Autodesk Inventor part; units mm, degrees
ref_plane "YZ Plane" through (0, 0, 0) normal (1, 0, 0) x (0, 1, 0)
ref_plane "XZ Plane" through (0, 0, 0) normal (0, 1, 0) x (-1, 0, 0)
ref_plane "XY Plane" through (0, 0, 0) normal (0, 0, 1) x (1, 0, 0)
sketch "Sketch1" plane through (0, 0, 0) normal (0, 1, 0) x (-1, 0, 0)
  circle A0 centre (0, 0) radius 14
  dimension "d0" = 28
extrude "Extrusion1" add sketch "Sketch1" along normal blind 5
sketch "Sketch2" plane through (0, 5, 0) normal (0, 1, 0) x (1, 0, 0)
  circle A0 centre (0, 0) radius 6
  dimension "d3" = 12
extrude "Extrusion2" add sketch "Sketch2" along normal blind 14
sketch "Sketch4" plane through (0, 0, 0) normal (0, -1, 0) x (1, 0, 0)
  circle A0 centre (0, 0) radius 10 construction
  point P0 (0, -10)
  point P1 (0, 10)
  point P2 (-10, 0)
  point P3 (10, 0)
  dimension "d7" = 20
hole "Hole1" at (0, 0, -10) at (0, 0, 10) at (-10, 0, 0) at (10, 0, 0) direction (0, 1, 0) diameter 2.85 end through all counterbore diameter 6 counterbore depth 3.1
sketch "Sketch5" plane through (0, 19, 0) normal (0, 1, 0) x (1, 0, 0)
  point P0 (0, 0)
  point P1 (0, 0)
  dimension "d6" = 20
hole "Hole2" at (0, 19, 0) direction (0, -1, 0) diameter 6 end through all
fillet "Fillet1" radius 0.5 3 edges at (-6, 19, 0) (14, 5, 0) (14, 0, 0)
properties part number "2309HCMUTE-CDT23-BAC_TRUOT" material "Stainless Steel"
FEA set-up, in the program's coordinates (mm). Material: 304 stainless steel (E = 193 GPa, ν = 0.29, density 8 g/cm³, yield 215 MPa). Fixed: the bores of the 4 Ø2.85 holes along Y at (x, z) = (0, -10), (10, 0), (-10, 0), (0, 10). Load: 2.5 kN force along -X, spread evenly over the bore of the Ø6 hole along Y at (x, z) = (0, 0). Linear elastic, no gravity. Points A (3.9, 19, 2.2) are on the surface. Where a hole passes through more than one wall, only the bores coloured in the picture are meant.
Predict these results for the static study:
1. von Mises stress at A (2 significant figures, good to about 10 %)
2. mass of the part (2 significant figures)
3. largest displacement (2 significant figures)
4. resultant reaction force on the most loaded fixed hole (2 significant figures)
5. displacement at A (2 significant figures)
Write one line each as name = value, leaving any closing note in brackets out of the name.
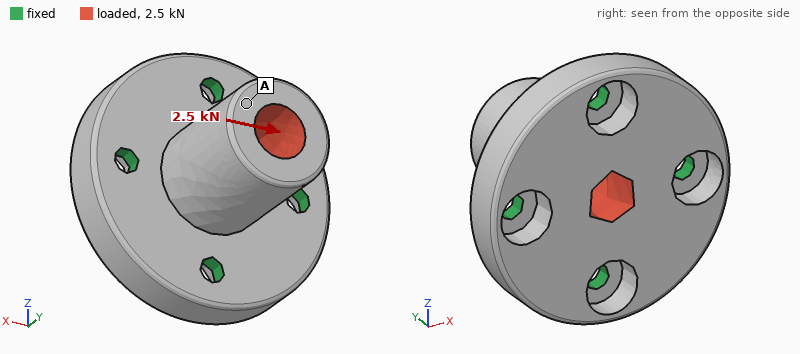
von Mises stress at A = 12 MPa
mass of the part = 30 g
largest displacement = 15 µm
resultant reaction force on the most loaded fixed hole = 960 N
displacement at A = 15 µm
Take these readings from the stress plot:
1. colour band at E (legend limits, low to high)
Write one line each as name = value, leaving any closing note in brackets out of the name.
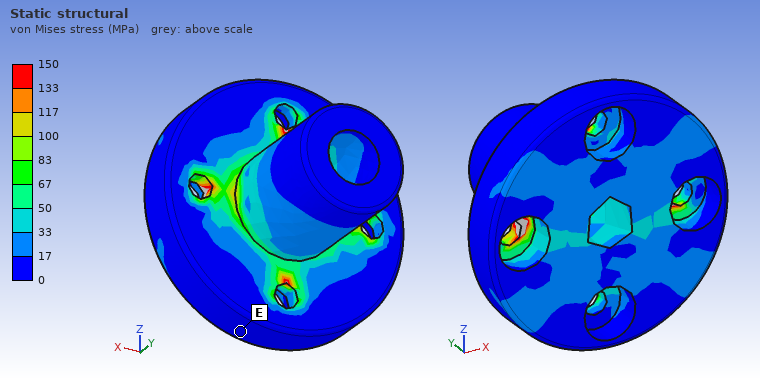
colour band at E = 0 to 17 MPa
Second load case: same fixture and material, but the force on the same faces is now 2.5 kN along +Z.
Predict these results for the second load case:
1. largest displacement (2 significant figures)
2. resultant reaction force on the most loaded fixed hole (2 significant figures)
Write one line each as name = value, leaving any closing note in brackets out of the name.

largest displacement = 15 µm
resultant reaction force on the most loaded fixed hole = 960 N
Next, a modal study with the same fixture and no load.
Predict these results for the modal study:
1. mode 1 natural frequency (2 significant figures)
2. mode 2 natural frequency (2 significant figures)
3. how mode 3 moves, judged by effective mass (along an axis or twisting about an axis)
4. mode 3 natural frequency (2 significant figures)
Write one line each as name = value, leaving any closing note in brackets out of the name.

mode 1 natural frequency = 21 kHz
mode 2 natural frequency = 21 kHz
how mode 3 moves, judged by effective mass = along Y
mode 3 natural frequency = 34 kHz
